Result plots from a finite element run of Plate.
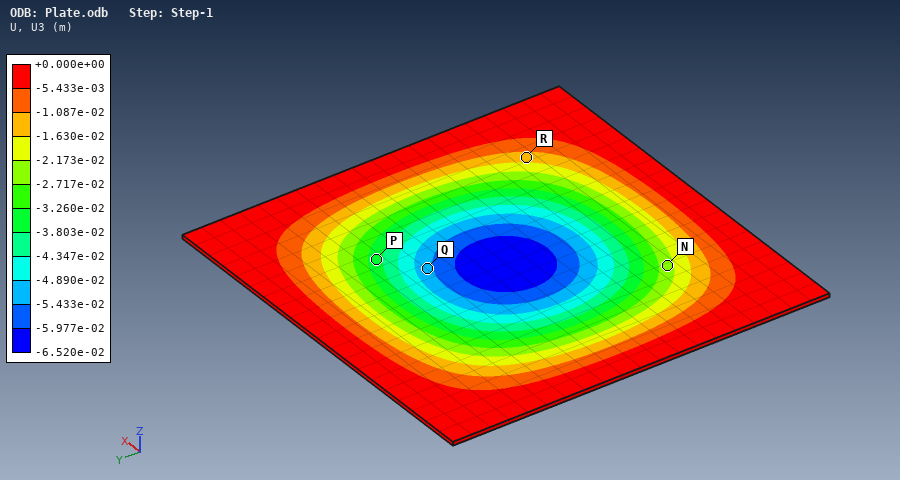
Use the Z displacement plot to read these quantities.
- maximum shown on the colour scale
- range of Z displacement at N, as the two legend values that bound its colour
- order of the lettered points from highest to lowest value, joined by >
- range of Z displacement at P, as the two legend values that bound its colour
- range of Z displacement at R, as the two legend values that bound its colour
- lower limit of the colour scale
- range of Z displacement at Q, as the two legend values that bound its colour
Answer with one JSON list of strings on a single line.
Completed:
["+0.000e+00 m", "-2.717e-02 to -2.173e-02 m", "R > N > P > Q", "-3.803e-02 to -3.260e-02 m", "-1.630e-02 to -1.087e-02 m", "-6.520e-02 m", "-5.433e-02 to -4.890e-02 m"]
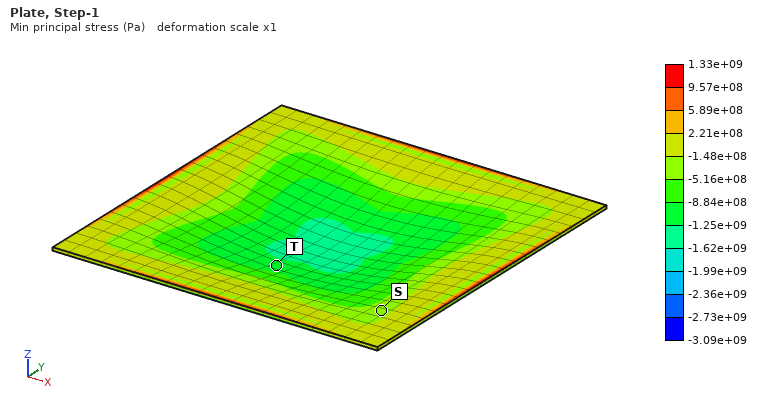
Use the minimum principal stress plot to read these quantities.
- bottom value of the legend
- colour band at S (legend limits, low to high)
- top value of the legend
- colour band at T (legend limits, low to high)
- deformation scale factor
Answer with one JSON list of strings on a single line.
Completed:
["-3.09e+09 Pa", "-5.16e+08 to -1.48e+08 Pa", "1.33e+09 Pa", "-1.25e+09 to -8.84e+08 Pa", "1"]
